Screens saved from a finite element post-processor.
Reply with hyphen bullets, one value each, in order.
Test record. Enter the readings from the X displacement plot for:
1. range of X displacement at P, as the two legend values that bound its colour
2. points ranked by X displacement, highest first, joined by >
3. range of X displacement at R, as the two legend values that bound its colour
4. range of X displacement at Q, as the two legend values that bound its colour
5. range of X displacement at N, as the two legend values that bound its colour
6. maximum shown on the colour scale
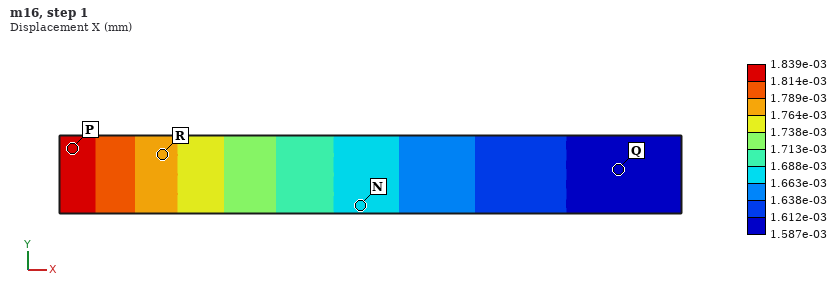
- 1.814e-03 to 1.839e-03 mm
- P > R > N > Q
- 1.764e-03 to 1.789e-03 mm
- 1.587e-03 to 1.612e-03 mm
- 1.663e-03 to 1.688e-03 mm
- 1.839e-03 mm
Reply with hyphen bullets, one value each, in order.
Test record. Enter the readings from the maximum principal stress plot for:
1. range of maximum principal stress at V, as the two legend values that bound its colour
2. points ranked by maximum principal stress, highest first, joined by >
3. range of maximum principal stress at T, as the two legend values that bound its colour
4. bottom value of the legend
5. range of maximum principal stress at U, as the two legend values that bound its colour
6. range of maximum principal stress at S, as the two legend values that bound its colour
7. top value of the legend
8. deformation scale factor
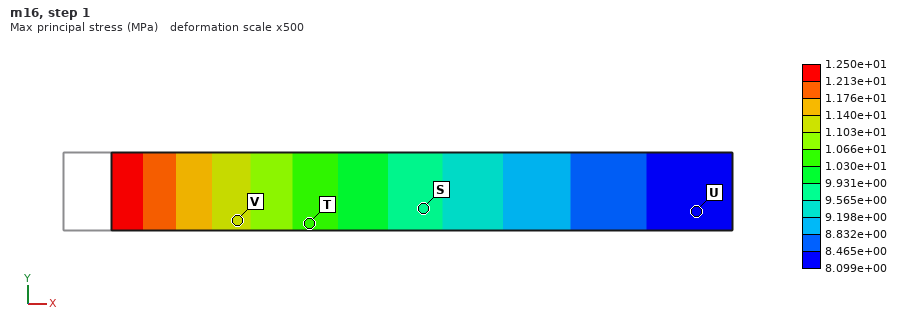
- 1.103e+01 to 1.140e+01 MPa
- V > T > S > U
- 1.030e+01 to 1.066e+01 MPa
- 8.099e+00 MPa
- 8.099e+00 to 8.465e+00 MPa
- 9.565e+00 to 9.931e+00 MPa
- 1.250e+01 MPa
- 500
